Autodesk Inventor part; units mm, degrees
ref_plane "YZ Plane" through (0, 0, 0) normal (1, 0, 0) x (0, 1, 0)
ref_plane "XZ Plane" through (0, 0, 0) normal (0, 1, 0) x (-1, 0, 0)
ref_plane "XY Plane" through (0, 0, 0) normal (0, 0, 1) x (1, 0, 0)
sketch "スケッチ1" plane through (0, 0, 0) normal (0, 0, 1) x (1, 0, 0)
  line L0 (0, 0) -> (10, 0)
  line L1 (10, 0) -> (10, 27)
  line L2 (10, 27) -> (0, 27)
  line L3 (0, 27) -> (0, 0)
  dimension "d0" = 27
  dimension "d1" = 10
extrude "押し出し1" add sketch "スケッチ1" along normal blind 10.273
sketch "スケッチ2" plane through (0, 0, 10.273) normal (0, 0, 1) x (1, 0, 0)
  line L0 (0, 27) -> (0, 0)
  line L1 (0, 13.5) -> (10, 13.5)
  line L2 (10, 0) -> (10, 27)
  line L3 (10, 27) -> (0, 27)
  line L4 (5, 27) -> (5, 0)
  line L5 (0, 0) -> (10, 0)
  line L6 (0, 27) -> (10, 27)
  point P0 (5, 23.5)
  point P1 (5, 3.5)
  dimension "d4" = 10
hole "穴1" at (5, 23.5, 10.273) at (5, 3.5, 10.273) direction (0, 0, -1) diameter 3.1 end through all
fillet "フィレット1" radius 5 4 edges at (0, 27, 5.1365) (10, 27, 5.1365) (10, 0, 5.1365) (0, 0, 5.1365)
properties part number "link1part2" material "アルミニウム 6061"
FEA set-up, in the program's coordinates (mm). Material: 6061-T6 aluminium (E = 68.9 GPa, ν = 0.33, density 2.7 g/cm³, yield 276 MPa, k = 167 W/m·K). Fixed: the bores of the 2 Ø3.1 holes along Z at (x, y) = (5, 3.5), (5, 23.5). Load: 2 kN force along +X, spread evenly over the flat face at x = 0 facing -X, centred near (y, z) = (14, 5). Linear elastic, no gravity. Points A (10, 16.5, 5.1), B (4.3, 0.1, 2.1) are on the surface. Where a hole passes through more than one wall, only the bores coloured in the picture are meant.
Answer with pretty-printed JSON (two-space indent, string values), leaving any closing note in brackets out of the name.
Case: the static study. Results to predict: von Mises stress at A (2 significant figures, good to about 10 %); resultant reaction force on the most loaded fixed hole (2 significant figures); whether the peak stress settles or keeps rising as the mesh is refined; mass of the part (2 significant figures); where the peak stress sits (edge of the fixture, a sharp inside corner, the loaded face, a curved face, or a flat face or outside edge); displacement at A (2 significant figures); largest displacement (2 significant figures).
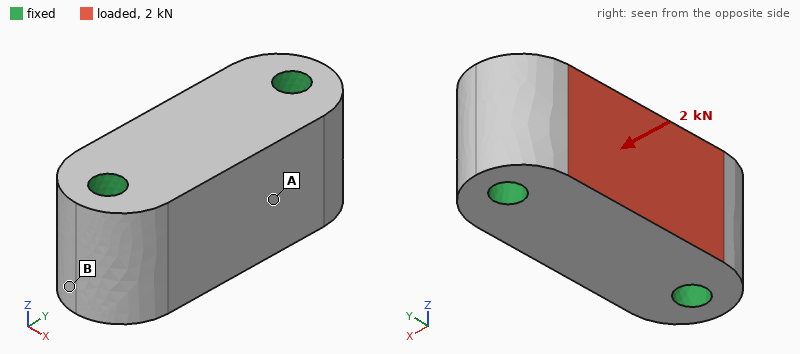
{
  "von Mises stress at A": "16 MPa",
  "resultant reaction force on the most loaded fixed hole": "1.0 kN",
  "whether the peak stress settles or keeps rising as the mesh is refined": "keeps rising",
  "mass of the part": "6.5 g",
  "where the peak stress sits": "edge of the fixture",
  "displacement at A": "2.9 µm",
  "largest displacement": "4.4 µm"
}
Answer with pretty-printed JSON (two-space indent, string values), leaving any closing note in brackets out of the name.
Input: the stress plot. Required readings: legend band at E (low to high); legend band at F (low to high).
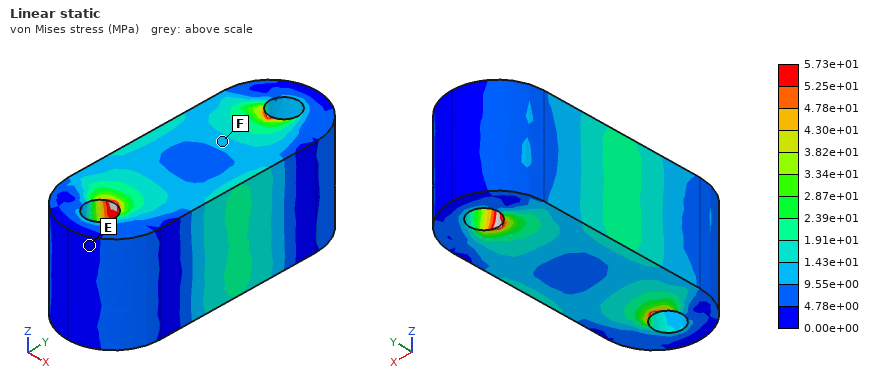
{
  "legend band at E": "0.00e+00 to 4.78e+00 MPa",
  "legend band at F": "9.55e+00 to 1.43e+01 MPa"
}
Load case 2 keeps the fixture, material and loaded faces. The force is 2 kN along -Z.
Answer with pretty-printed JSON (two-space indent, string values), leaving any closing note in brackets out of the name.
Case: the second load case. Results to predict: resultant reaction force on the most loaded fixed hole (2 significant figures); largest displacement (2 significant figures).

{
  "resultant reaction force on the most loaded fixed hole": "1.0 kN",
  "largest displacement": "9.7 µm"
}
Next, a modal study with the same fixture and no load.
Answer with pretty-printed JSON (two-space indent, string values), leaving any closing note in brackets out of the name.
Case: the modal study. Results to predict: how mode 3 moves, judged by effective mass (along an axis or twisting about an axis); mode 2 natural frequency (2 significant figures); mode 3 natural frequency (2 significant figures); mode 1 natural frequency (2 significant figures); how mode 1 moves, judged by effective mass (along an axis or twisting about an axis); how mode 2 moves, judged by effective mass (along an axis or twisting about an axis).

{
  "how mode 3 moves, judged by effective mass": "twisting about Y",
  "mode 2 natural frequency": "65 kHz",
  "mode 3 natural frequency": "72 kHz",
  "mode 1 natural frequency": "58 kHz",
  "how mode 1 moves, judged by effective mass": "along X",
  "how mode 2 moves, judged by effective mass": "along Z"
}
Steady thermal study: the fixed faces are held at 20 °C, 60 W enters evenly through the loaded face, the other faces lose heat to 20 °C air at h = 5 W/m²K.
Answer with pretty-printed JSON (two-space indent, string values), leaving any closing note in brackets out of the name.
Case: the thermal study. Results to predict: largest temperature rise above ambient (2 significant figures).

{
  "largest temperature rise above ambient": "16 K"
}
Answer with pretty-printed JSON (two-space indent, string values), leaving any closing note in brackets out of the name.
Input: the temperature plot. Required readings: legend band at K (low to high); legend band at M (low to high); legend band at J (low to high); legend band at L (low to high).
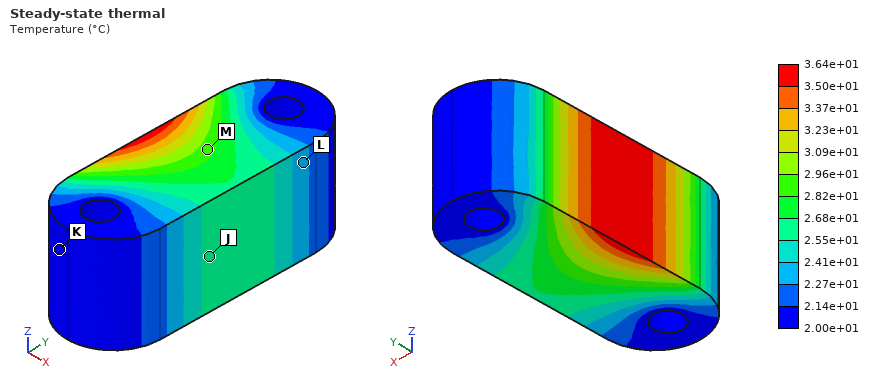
{
  "legend band at K": "2.00e+01 to 2.14e+01 °C",
  "legend band at M": "2.82e+01 to 2.96e+01 °C",
  "legend band at J": "2.55e+01 to 2.68e+01 °C",
  "legend band at L": "2.27e+01 to 2.41e+01 °C"
}
